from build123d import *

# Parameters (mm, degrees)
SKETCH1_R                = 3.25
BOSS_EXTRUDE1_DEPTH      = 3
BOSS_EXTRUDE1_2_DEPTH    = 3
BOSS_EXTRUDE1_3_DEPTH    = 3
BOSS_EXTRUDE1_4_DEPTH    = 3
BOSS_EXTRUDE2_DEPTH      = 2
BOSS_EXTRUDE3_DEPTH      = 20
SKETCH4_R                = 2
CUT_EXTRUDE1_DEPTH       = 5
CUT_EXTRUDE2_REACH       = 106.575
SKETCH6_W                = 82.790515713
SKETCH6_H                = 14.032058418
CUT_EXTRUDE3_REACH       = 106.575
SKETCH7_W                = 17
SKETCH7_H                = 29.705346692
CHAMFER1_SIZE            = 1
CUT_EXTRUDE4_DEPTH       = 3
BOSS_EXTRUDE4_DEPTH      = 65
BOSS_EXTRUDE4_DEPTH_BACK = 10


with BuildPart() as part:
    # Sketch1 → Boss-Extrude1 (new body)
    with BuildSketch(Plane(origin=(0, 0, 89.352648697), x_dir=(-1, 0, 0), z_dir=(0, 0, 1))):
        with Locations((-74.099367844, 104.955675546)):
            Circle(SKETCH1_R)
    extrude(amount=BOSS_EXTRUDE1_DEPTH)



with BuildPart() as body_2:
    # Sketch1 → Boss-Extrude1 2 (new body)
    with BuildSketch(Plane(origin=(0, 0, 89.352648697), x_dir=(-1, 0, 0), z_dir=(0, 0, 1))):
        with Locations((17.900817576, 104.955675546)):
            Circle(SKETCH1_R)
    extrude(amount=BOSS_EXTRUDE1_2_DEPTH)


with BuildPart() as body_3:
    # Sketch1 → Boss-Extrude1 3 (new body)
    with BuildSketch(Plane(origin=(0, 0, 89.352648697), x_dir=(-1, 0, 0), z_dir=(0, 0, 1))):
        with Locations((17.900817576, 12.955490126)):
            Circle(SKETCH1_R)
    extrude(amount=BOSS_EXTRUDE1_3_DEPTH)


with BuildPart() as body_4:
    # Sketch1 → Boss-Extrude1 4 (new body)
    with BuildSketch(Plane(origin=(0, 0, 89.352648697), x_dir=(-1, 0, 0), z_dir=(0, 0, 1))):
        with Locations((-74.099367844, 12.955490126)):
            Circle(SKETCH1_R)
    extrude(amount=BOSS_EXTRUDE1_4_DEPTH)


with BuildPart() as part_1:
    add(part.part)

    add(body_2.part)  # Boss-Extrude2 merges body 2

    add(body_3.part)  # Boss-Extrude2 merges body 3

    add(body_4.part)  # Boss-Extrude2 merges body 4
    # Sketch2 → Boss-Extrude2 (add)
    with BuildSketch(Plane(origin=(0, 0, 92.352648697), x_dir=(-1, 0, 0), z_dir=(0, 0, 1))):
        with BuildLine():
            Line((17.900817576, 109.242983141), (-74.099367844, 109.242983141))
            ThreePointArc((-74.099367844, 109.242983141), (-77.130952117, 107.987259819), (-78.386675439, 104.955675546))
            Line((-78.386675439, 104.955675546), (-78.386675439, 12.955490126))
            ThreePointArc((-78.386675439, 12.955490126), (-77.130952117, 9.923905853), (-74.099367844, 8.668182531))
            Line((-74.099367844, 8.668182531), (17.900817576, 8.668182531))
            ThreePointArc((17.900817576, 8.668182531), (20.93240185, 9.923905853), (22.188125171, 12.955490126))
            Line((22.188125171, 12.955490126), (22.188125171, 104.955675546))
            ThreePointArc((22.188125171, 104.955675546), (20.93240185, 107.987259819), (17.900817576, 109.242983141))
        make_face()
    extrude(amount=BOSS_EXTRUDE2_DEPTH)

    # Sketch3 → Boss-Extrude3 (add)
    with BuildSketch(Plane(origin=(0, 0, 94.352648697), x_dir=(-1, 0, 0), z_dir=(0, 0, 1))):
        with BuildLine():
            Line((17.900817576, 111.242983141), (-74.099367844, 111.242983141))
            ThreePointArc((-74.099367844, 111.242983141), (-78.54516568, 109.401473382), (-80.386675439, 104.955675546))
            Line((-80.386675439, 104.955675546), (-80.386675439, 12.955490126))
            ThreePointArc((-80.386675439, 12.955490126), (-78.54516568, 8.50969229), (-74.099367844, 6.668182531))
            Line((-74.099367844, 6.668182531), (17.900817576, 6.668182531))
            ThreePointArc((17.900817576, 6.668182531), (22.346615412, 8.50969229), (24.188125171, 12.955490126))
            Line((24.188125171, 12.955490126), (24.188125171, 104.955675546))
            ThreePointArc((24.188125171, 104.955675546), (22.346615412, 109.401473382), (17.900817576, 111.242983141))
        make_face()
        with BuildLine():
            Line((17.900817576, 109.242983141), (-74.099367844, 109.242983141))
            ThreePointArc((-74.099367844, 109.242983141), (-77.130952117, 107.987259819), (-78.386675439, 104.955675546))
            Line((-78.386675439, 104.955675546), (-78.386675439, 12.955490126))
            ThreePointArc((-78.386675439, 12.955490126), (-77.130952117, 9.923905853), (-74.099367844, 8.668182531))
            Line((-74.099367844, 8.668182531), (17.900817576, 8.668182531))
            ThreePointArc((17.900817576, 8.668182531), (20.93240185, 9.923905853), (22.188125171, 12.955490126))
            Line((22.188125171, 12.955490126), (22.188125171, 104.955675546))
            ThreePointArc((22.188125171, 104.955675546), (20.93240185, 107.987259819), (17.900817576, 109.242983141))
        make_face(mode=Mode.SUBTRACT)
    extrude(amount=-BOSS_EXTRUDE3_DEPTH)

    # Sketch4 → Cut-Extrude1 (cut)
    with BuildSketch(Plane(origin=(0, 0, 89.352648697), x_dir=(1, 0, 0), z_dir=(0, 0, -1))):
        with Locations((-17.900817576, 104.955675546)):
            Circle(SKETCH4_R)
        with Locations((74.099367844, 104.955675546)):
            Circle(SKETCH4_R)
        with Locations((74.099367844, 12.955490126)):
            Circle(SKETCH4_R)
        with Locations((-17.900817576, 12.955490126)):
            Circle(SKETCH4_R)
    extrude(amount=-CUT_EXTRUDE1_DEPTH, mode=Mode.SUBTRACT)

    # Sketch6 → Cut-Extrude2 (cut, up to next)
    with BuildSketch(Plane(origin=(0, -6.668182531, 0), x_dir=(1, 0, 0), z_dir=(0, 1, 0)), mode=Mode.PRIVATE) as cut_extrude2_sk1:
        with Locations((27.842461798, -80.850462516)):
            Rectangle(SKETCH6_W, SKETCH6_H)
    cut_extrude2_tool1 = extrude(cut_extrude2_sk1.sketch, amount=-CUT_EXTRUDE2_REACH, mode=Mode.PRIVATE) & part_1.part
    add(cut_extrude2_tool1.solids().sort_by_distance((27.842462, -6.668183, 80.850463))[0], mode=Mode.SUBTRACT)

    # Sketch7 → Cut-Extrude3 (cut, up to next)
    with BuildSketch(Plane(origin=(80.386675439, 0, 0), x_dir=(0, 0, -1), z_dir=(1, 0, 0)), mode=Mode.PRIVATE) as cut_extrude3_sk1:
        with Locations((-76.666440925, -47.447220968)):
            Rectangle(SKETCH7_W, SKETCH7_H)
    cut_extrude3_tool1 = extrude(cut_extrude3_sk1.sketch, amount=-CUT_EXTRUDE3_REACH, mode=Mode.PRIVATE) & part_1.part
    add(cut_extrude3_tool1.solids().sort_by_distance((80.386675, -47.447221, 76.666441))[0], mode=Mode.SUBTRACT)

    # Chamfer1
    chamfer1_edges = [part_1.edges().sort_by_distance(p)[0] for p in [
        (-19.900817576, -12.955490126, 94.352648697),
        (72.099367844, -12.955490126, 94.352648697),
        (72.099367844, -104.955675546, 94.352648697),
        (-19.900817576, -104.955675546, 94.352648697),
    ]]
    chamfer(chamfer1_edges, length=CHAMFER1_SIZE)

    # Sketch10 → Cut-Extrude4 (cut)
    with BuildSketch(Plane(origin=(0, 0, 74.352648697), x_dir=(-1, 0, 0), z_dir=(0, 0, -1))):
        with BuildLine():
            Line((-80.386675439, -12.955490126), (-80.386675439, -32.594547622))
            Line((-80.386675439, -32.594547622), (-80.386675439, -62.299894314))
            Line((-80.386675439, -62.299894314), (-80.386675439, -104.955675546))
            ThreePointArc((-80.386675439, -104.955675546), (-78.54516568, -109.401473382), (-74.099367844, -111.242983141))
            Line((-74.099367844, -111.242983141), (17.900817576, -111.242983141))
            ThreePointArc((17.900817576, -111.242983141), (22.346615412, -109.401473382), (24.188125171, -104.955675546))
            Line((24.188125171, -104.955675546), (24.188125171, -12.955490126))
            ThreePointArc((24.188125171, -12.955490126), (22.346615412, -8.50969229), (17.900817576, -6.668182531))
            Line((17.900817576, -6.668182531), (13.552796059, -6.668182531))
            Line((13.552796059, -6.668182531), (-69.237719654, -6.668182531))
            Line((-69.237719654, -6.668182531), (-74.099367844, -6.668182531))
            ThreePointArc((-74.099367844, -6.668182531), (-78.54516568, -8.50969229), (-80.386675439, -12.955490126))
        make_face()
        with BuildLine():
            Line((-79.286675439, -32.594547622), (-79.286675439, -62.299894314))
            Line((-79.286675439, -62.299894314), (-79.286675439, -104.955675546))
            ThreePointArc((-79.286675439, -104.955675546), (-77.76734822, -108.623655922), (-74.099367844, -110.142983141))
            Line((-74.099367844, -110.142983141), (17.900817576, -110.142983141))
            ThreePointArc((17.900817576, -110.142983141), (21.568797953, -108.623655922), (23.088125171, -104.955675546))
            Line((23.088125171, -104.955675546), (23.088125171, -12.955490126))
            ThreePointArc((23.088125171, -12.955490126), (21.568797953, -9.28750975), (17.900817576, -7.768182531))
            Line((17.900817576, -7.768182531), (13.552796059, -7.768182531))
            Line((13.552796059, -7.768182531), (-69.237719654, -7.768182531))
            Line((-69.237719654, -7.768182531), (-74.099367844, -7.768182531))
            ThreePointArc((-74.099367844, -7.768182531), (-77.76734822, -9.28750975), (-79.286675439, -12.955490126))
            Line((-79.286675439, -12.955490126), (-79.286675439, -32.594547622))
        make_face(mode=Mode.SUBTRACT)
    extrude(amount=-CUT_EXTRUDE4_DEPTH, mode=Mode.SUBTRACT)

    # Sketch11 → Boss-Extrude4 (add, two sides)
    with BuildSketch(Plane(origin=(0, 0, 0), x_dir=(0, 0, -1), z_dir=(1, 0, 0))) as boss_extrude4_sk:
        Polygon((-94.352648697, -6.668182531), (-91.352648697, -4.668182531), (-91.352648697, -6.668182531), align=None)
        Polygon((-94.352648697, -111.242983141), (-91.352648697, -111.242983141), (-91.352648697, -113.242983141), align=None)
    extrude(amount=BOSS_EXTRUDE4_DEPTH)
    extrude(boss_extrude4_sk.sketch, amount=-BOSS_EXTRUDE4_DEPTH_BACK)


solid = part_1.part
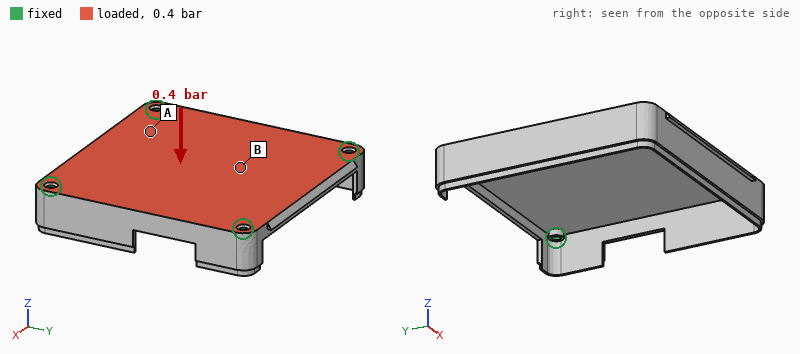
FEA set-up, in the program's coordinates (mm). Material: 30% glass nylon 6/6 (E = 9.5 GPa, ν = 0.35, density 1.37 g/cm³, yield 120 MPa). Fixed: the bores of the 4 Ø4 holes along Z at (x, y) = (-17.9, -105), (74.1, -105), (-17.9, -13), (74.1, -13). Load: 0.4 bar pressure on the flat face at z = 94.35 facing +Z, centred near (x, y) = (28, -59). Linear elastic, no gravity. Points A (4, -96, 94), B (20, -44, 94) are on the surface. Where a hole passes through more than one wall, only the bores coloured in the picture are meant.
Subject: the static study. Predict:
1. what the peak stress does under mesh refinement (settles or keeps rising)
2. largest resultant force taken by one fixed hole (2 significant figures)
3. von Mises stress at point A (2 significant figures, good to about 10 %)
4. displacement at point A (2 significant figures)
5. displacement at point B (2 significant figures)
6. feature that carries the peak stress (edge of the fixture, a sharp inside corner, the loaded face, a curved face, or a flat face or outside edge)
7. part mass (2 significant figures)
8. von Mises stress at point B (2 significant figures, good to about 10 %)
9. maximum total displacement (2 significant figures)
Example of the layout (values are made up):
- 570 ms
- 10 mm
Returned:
- keeps rising
- 110 N
- 12 MPa
- 0.49 mm
- 1.6 mm
- edge of the fixture
- 45 g
- 22 MPa
- 1.8 mm
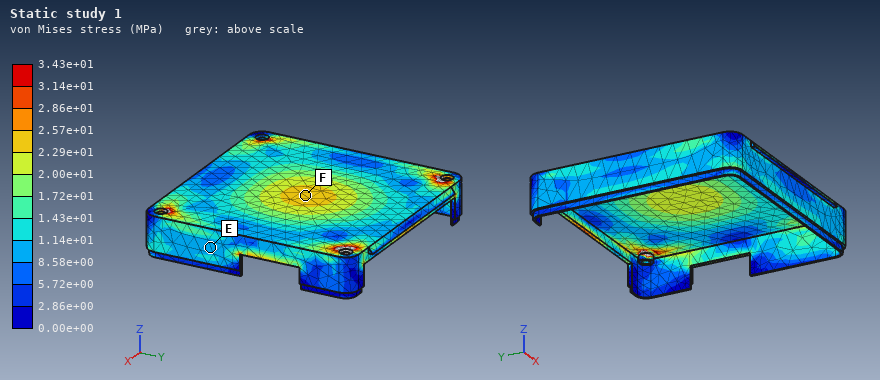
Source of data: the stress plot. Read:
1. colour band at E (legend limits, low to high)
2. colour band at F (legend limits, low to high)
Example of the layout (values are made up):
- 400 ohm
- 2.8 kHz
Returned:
- 8.58e+00 to 1.14e+01 MPa
- 2.29e+01 to 2.57e+01 MPa
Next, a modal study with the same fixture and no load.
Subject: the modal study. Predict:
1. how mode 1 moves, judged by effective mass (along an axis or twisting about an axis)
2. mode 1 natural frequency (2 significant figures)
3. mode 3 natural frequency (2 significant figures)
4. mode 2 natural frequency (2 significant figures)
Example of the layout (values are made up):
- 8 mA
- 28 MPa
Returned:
- along Z
- 560 Hz
- 1200 Hz
- 1100 Hz
